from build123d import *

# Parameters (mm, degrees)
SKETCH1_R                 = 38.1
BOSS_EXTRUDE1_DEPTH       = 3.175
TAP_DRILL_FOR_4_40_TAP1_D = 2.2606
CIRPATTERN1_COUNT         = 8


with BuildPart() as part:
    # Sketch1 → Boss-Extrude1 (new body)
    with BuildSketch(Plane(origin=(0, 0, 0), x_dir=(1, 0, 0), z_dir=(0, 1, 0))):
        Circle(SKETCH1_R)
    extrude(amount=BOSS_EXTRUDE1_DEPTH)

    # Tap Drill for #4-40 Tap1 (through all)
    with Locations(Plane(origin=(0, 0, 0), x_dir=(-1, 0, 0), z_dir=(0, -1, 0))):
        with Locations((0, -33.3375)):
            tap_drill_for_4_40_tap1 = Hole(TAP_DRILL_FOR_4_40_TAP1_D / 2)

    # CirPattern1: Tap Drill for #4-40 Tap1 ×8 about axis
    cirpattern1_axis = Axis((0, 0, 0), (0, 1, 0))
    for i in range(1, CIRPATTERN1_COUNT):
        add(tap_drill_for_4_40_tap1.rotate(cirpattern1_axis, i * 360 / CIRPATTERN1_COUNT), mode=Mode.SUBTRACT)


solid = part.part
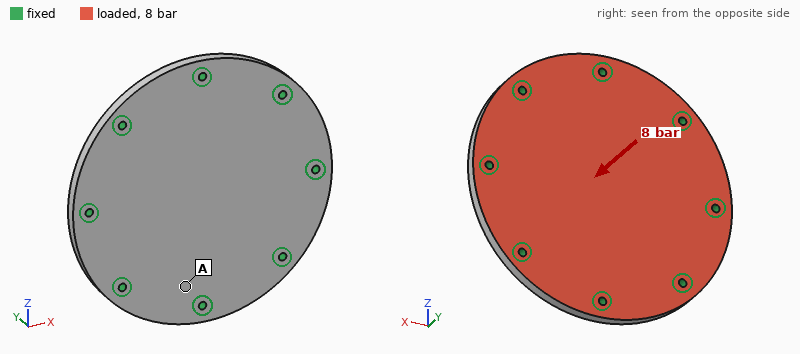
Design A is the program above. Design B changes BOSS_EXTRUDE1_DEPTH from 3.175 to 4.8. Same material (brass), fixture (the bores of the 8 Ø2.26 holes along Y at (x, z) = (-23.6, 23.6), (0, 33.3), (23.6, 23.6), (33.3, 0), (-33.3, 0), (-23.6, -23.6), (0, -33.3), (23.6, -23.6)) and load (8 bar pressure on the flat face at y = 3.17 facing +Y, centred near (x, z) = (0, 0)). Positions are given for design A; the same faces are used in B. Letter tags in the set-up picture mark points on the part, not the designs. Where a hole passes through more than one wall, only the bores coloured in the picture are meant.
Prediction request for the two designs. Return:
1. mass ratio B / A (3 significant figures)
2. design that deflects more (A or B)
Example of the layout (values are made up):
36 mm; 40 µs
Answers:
1.51; A
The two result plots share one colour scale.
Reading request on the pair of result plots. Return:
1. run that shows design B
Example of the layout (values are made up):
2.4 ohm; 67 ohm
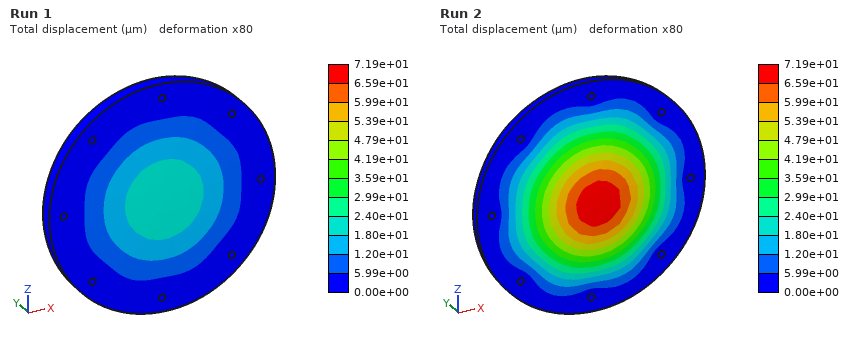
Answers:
Run 1
